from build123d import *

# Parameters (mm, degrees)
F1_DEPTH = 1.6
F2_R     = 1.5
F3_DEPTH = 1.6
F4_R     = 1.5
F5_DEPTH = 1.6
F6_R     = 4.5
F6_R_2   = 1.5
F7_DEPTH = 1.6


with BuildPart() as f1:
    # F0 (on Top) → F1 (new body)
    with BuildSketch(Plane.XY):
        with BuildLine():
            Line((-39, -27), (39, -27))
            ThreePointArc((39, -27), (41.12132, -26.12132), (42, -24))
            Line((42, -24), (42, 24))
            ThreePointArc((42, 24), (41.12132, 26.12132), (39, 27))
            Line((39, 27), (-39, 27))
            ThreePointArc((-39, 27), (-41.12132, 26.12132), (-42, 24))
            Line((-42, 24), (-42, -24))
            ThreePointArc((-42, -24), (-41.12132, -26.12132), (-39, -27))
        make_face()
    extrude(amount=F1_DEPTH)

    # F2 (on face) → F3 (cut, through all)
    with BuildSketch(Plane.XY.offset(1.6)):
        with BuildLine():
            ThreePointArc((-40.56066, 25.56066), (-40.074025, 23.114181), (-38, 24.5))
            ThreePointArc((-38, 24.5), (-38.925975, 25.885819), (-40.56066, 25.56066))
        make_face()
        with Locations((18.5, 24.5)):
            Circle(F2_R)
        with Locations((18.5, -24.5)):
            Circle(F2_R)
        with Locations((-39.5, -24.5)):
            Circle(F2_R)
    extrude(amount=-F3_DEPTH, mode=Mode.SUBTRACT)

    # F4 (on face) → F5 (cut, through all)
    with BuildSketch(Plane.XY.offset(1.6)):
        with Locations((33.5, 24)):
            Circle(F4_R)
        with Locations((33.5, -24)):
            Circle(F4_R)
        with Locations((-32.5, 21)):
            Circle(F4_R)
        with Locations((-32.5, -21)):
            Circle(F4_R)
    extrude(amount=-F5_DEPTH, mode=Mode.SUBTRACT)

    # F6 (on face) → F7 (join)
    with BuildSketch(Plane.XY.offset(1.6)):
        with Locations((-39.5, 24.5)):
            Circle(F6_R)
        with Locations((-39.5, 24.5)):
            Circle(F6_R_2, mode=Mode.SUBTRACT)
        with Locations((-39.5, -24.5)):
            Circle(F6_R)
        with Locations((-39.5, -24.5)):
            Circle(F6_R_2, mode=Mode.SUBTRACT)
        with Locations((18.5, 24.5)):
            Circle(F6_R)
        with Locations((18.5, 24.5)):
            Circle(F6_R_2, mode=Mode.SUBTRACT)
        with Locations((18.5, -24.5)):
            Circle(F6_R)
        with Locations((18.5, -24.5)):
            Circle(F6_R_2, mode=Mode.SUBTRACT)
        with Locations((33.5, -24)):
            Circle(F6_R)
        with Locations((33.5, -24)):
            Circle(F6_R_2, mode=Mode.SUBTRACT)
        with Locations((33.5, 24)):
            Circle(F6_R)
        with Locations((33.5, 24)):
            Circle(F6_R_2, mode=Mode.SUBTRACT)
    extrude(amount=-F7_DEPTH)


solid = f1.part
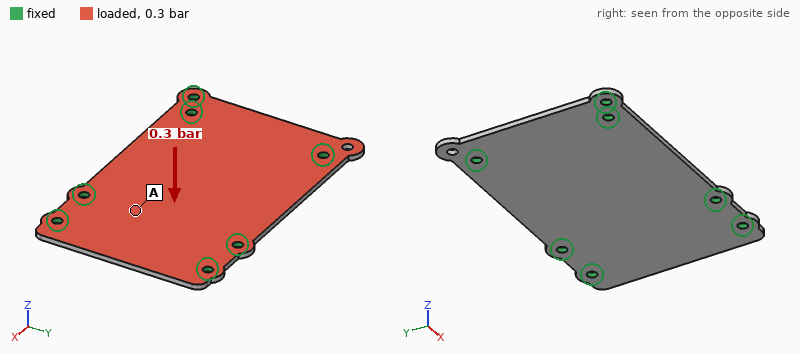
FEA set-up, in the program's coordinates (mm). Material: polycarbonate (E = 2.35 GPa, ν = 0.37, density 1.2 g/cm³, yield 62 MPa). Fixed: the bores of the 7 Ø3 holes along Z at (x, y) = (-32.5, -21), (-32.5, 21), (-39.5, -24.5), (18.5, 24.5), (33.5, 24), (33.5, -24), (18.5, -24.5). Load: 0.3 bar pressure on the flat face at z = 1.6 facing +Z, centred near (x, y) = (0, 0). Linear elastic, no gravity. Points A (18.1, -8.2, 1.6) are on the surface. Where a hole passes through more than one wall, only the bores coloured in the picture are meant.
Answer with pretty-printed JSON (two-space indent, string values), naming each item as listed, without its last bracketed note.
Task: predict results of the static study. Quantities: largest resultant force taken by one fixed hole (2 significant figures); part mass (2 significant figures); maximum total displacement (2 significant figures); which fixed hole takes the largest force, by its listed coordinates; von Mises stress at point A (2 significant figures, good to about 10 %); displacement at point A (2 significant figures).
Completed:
{
  "largest resultant force taken by one fixed hole": "33 N",
  "part mass": "8.7 g",
  "maximum total displacement": "1.2 mm",
  "which fixed hole takes the largest force, by its listed coordinates": "(-32.5, -21)",
  "von Mises stress at point A": "6.2 MPa",
  "displacement at point A": "0.58 mm"
}
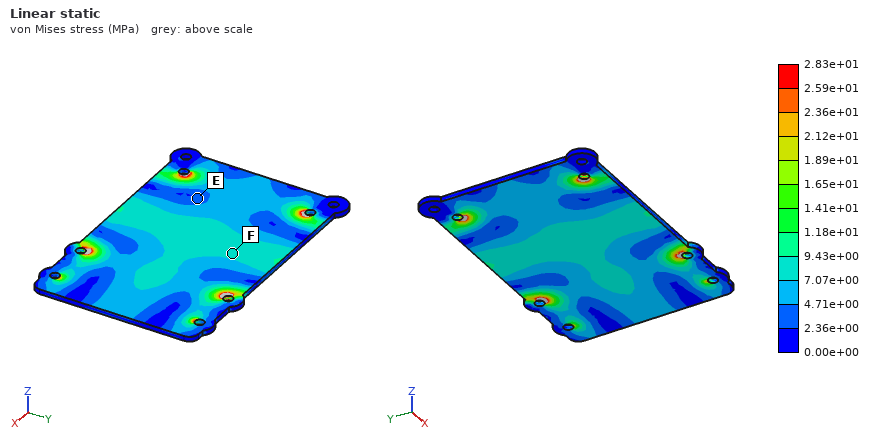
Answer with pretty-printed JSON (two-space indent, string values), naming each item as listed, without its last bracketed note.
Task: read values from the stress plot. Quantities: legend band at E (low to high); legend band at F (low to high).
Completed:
{
  "legend band at E": "2.36e+00 to 4.71e+00 MPa",
  "legend band at F": "7.07e+00 to 9.43e+00 MPa"
}
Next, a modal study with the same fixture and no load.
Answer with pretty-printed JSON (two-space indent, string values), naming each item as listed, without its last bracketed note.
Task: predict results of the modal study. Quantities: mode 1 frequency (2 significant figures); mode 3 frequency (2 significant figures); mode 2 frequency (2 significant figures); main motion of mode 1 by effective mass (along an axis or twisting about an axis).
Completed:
{
  "mode 1 frequency": "700 Hz",
  "mode 3 frequency": "1100 Hz",
  "mode 2 frequency": "1100 Hz",
  "main motion of mode 1 by effective mass": "along Z"
}
